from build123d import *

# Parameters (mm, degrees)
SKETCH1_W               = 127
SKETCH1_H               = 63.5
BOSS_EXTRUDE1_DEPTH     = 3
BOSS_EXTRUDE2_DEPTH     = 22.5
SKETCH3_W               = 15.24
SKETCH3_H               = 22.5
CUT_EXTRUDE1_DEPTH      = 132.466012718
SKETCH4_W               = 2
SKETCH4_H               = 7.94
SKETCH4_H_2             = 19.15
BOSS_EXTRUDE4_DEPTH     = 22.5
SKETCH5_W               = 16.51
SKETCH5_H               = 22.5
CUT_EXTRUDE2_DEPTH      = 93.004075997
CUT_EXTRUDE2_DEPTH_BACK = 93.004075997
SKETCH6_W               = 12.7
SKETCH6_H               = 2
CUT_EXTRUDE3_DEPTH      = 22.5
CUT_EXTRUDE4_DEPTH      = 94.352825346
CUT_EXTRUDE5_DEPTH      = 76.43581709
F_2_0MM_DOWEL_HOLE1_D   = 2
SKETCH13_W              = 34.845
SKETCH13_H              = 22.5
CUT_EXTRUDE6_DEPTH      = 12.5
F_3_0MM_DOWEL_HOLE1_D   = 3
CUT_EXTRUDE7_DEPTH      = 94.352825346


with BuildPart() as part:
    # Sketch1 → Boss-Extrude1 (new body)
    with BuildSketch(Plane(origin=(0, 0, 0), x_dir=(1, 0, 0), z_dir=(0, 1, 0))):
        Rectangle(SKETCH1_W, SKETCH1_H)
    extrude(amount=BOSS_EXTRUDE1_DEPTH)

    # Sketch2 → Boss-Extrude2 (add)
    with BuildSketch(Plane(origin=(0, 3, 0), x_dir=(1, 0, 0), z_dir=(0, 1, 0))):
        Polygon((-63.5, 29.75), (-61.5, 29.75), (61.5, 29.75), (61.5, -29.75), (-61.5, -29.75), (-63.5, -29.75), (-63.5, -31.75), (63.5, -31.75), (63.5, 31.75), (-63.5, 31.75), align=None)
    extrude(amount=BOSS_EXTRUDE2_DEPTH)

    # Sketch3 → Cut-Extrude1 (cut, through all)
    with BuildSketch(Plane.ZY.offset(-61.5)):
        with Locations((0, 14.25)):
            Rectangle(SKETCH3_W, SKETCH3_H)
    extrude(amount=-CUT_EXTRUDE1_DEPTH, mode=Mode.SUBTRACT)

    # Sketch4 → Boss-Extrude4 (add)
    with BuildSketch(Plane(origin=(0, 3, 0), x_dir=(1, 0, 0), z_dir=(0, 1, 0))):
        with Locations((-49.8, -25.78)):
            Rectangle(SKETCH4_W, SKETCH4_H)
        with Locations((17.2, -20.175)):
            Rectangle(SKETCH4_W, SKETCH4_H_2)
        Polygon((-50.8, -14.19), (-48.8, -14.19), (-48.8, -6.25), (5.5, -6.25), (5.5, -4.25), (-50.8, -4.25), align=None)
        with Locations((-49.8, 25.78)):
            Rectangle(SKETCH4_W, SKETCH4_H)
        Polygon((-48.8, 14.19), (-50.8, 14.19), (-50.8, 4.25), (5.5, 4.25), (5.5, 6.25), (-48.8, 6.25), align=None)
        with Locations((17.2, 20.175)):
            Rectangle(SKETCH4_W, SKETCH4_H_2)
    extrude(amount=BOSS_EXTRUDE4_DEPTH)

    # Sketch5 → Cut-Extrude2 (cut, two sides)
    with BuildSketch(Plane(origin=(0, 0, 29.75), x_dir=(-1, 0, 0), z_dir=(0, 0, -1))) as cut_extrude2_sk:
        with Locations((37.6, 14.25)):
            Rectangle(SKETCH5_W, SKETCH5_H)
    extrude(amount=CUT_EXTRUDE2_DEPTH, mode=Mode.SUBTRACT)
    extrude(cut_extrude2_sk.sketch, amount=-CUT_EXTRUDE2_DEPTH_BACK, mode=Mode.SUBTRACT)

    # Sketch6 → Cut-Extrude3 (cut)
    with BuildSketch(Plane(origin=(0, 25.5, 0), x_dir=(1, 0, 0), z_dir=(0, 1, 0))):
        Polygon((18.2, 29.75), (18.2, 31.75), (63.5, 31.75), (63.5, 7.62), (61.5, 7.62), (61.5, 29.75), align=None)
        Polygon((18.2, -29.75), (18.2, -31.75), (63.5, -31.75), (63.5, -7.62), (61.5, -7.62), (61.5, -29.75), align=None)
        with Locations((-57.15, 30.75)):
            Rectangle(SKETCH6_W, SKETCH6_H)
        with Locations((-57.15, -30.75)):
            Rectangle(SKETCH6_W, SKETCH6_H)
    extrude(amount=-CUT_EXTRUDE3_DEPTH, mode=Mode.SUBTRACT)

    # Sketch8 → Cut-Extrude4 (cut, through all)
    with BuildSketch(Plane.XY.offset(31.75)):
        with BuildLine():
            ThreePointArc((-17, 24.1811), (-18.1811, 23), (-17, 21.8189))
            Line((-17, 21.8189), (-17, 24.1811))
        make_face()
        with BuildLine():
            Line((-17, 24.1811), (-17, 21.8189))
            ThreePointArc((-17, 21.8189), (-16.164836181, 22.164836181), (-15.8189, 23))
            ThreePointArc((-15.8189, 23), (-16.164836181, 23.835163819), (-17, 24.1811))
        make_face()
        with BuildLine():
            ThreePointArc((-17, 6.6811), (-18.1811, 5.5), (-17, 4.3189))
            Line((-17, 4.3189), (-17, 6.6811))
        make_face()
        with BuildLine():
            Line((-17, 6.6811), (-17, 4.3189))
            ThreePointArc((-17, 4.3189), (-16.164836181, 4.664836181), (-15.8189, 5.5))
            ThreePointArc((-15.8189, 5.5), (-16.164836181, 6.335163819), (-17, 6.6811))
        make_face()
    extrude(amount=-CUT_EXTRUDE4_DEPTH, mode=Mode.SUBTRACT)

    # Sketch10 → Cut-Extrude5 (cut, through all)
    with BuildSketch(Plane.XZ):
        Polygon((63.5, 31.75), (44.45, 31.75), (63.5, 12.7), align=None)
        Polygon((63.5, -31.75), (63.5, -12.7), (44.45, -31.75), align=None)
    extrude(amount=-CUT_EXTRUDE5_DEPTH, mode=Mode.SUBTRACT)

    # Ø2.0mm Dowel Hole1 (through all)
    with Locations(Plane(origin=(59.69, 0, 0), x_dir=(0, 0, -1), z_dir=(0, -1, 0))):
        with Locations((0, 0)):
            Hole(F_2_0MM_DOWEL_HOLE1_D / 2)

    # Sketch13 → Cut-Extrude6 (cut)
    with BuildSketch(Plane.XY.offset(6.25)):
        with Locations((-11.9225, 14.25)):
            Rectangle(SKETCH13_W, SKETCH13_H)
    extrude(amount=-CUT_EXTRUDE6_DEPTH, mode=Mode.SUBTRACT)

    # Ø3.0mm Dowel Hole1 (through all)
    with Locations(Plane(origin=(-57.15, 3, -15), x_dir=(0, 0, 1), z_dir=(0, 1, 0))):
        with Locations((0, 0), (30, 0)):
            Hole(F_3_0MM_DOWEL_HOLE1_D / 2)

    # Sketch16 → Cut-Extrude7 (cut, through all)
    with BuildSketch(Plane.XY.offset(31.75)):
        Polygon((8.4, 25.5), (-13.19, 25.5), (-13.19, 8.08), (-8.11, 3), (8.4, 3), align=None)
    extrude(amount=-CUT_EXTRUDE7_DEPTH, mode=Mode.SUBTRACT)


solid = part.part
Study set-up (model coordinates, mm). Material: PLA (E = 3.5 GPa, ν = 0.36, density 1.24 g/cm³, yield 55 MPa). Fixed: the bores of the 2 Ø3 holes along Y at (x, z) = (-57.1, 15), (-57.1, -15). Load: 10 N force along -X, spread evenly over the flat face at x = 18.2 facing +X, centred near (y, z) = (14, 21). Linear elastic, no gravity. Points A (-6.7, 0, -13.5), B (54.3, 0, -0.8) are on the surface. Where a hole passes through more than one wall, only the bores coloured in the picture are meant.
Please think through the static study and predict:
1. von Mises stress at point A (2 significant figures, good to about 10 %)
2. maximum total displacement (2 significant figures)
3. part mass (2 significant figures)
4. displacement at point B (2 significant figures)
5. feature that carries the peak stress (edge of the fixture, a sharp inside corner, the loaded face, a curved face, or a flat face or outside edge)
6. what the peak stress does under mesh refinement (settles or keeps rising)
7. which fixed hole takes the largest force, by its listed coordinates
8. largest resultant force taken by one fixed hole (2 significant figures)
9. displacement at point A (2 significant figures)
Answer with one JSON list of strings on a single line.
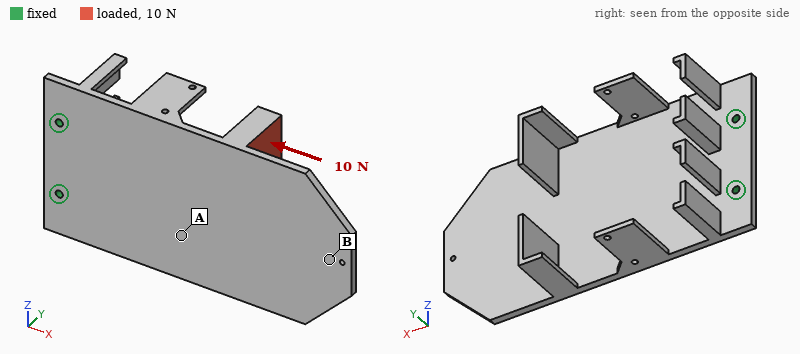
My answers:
["1.1 MPa", "1.5 mm", "37 g", "1.3 mm", "edge of the fixture", "keeps rising", "(-57.1, 15)", "12 N", "0.32 mm"]
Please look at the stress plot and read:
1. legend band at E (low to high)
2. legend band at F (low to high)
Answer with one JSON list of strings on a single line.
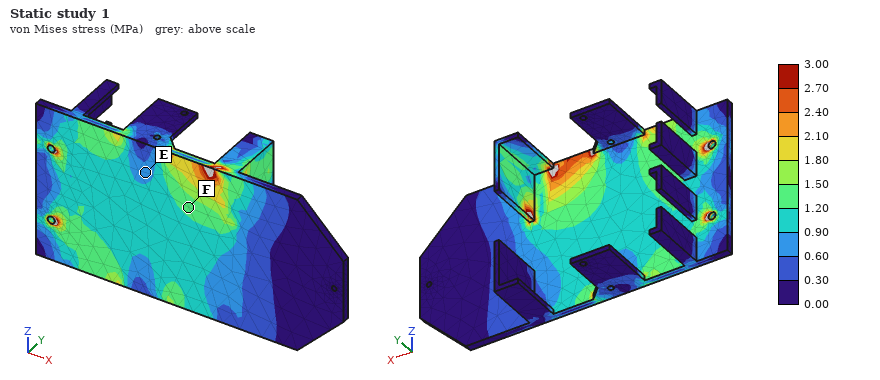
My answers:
["0.60 to 0.90 MPa", "1.20 to 1.50 MPa"]
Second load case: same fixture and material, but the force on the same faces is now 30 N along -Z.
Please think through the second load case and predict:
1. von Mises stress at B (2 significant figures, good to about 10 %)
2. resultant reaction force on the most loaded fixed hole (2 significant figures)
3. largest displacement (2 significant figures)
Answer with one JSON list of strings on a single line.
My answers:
["0.89 MPa", "74 N", "1.3 mm"]
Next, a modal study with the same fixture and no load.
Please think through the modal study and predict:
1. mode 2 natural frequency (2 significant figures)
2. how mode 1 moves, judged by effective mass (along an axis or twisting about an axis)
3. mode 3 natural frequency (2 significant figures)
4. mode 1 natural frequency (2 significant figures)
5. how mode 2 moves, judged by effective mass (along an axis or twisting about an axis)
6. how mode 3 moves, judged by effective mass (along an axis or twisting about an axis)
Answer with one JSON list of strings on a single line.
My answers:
["200 Hz", "along Y", "330 Hz", "58 Hz", "twisting about X", "along Y"]
